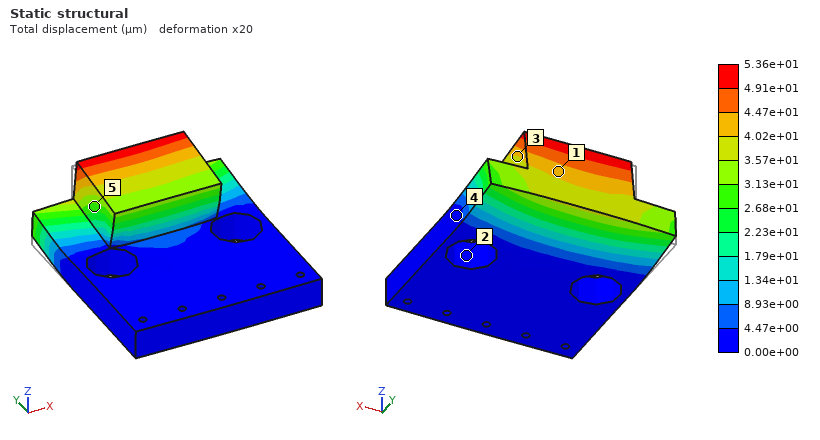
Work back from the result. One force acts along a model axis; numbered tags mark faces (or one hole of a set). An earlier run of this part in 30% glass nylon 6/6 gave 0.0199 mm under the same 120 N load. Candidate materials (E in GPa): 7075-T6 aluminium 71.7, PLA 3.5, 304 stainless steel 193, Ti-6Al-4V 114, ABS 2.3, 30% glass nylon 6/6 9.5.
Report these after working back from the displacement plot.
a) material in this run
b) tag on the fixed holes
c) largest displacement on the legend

PLA
2
5.36e+01 µm
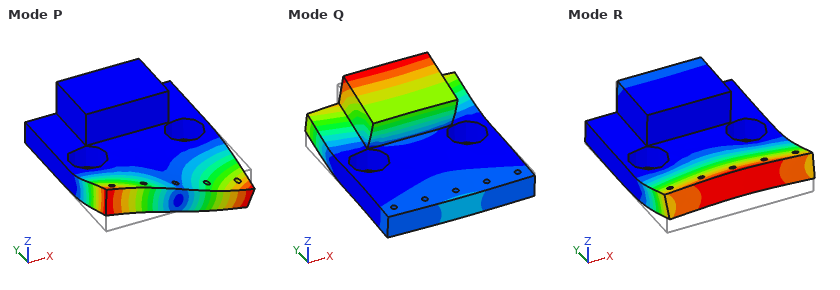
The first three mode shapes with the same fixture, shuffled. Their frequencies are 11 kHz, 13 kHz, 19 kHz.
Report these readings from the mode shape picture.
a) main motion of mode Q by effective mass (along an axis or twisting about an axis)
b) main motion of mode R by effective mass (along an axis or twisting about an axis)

along Z
along Z
